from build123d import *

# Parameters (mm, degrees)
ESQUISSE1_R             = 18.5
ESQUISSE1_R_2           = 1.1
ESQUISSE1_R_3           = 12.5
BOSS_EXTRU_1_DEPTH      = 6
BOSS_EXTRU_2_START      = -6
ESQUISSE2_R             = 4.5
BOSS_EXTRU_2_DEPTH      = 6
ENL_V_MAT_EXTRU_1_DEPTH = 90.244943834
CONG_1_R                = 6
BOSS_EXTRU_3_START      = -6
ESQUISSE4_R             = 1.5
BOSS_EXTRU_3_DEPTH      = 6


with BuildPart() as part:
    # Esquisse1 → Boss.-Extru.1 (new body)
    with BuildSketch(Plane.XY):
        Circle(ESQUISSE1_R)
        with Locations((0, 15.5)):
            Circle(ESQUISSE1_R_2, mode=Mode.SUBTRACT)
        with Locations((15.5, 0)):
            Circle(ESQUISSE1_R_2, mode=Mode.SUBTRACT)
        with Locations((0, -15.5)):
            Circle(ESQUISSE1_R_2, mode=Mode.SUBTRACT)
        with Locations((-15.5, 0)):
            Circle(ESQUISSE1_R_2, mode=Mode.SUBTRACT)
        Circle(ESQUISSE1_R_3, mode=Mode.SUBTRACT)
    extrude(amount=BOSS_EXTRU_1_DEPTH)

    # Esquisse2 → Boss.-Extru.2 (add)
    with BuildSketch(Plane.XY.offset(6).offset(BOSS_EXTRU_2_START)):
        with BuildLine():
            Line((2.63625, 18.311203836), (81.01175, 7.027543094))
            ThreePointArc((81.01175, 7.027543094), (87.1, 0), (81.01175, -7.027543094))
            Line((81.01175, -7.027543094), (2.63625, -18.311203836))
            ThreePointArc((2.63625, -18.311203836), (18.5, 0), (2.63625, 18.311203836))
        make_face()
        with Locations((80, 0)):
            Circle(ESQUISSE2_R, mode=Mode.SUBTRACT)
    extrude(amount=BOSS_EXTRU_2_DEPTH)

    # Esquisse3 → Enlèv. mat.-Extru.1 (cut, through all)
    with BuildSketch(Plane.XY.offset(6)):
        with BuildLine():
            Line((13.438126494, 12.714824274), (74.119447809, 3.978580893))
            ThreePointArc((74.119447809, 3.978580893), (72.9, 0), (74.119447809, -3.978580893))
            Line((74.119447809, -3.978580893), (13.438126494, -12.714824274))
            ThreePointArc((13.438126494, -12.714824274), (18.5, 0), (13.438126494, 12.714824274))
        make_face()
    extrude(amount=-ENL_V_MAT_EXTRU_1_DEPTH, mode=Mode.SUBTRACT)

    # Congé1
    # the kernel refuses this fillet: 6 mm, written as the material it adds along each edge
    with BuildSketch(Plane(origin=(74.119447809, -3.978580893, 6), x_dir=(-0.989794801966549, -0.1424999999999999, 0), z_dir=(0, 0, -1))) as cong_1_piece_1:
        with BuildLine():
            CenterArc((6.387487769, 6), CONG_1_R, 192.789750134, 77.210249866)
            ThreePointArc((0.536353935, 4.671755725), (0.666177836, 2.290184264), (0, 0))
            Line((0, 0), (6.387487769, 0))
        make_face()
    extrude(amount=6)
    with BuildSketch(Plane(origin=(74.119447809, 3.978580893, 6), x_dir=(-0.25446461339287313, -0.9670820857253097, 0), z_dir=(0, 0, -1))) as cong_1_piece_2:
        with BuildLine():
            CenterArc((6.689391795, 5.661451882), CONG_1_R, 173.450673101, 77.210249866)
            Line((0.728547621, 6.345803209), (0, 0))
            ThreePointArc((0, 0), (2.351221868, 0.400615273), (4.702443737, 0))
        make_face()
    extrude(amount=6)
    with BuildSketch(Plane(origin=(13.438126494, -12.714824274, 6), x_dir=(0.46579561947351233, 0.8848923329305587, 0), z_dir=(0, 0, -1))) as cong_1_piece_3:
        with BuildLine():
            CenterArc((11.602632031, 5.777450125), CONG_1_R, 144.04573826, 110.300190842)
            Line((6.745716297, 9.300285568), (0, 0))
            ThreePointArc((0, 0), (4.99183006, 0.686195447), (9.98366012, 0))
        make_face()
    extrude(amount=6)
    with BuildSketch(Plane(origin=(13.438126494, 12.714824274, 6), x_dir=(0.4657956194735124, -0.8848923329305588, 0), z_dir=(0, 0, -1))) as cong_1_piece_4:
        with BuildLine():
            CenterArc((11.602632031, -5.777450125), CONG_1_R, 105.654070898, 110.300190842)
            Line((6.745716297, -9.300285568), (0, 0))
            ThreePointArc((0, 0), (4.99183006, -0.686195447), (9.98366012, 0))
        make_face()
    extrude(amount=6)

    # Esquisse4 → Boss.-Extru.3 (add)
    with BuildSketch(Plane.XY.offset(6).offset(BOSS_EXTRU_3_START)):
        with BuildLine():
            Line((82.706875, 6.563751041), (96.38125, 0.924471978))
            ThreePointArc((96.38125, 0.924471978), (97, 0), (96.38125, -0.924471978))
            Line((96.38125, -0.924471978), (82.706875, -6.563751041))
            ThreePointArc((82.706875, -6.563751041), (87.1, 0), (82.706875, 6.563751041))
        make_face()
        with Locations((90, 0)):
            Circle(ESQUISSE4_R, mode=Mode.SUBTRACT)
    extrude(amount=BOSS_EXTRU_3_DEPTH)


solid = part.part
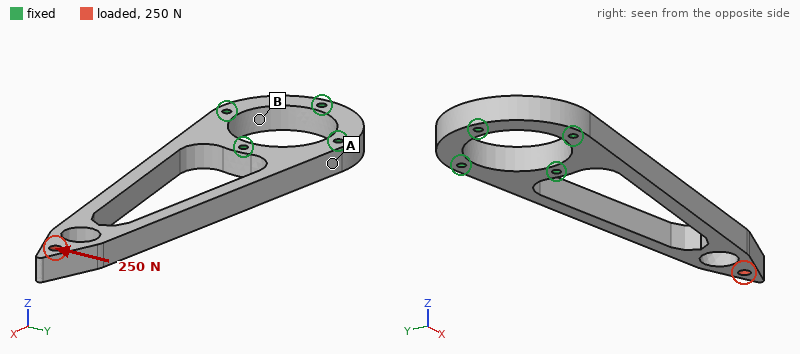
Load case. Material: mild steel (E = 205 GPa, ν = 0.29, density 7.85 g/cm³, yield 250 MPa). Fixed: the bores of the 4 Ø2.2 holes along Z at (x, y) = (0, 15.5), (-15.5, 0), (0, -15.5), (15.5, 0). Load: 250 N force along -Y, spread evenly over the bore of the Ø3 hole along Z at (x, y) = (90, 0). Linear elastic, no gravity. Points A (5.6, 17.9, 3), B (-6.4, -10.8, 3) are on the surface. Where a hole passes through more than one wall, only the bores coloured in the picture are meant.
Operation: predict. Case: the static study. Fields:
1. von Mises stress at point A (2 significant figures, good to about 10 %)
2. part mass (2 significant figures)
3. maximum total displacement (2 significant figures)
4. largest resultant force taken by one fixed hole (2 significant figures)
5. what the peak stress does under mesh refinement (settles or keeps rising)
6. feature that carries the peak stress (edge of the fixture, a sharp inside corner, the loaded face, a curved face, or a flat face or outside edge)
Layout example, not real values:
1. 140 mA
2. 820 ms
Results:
1. 20 MPa
2. 62 g
3. 81 µm
4. 600 N
5. keeps rising
6. a sharp inside corner
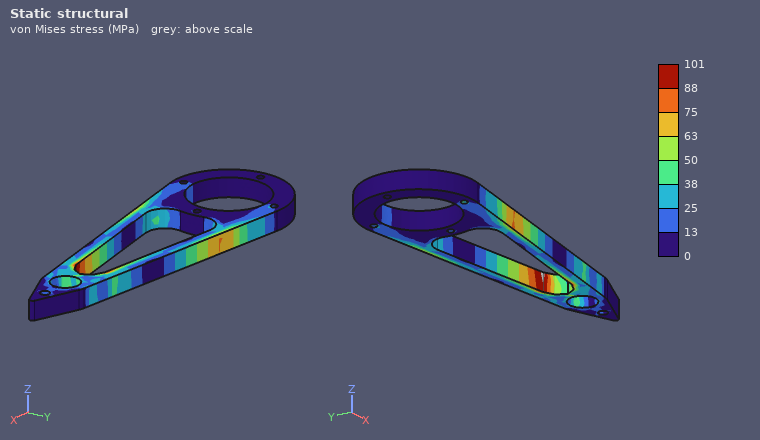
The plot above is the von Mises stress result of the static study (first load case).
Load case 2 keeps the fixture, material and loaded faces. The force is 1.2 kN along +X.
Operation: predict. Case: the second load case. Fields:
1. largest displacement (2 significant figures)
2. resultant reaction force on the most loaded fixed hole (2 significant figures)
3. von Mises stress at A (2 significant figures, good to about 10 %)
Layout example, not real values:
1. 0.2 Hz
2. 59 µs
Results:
1. 12 µm
2. 550 N
3. 17 MPa
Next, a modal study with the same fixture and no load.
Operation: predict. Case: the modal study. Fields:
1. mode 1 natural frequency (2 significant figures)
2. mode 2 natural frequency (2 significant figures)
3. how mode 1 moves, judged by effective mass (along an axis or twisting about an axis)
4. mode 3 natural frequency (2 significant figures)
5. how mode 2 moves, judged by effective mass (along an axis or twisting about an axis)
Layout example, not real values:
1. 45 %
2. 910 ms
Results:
1. 760 Hz
2. 1900 Hz
3. along Z
4. 3600 Hz
5. along Y
